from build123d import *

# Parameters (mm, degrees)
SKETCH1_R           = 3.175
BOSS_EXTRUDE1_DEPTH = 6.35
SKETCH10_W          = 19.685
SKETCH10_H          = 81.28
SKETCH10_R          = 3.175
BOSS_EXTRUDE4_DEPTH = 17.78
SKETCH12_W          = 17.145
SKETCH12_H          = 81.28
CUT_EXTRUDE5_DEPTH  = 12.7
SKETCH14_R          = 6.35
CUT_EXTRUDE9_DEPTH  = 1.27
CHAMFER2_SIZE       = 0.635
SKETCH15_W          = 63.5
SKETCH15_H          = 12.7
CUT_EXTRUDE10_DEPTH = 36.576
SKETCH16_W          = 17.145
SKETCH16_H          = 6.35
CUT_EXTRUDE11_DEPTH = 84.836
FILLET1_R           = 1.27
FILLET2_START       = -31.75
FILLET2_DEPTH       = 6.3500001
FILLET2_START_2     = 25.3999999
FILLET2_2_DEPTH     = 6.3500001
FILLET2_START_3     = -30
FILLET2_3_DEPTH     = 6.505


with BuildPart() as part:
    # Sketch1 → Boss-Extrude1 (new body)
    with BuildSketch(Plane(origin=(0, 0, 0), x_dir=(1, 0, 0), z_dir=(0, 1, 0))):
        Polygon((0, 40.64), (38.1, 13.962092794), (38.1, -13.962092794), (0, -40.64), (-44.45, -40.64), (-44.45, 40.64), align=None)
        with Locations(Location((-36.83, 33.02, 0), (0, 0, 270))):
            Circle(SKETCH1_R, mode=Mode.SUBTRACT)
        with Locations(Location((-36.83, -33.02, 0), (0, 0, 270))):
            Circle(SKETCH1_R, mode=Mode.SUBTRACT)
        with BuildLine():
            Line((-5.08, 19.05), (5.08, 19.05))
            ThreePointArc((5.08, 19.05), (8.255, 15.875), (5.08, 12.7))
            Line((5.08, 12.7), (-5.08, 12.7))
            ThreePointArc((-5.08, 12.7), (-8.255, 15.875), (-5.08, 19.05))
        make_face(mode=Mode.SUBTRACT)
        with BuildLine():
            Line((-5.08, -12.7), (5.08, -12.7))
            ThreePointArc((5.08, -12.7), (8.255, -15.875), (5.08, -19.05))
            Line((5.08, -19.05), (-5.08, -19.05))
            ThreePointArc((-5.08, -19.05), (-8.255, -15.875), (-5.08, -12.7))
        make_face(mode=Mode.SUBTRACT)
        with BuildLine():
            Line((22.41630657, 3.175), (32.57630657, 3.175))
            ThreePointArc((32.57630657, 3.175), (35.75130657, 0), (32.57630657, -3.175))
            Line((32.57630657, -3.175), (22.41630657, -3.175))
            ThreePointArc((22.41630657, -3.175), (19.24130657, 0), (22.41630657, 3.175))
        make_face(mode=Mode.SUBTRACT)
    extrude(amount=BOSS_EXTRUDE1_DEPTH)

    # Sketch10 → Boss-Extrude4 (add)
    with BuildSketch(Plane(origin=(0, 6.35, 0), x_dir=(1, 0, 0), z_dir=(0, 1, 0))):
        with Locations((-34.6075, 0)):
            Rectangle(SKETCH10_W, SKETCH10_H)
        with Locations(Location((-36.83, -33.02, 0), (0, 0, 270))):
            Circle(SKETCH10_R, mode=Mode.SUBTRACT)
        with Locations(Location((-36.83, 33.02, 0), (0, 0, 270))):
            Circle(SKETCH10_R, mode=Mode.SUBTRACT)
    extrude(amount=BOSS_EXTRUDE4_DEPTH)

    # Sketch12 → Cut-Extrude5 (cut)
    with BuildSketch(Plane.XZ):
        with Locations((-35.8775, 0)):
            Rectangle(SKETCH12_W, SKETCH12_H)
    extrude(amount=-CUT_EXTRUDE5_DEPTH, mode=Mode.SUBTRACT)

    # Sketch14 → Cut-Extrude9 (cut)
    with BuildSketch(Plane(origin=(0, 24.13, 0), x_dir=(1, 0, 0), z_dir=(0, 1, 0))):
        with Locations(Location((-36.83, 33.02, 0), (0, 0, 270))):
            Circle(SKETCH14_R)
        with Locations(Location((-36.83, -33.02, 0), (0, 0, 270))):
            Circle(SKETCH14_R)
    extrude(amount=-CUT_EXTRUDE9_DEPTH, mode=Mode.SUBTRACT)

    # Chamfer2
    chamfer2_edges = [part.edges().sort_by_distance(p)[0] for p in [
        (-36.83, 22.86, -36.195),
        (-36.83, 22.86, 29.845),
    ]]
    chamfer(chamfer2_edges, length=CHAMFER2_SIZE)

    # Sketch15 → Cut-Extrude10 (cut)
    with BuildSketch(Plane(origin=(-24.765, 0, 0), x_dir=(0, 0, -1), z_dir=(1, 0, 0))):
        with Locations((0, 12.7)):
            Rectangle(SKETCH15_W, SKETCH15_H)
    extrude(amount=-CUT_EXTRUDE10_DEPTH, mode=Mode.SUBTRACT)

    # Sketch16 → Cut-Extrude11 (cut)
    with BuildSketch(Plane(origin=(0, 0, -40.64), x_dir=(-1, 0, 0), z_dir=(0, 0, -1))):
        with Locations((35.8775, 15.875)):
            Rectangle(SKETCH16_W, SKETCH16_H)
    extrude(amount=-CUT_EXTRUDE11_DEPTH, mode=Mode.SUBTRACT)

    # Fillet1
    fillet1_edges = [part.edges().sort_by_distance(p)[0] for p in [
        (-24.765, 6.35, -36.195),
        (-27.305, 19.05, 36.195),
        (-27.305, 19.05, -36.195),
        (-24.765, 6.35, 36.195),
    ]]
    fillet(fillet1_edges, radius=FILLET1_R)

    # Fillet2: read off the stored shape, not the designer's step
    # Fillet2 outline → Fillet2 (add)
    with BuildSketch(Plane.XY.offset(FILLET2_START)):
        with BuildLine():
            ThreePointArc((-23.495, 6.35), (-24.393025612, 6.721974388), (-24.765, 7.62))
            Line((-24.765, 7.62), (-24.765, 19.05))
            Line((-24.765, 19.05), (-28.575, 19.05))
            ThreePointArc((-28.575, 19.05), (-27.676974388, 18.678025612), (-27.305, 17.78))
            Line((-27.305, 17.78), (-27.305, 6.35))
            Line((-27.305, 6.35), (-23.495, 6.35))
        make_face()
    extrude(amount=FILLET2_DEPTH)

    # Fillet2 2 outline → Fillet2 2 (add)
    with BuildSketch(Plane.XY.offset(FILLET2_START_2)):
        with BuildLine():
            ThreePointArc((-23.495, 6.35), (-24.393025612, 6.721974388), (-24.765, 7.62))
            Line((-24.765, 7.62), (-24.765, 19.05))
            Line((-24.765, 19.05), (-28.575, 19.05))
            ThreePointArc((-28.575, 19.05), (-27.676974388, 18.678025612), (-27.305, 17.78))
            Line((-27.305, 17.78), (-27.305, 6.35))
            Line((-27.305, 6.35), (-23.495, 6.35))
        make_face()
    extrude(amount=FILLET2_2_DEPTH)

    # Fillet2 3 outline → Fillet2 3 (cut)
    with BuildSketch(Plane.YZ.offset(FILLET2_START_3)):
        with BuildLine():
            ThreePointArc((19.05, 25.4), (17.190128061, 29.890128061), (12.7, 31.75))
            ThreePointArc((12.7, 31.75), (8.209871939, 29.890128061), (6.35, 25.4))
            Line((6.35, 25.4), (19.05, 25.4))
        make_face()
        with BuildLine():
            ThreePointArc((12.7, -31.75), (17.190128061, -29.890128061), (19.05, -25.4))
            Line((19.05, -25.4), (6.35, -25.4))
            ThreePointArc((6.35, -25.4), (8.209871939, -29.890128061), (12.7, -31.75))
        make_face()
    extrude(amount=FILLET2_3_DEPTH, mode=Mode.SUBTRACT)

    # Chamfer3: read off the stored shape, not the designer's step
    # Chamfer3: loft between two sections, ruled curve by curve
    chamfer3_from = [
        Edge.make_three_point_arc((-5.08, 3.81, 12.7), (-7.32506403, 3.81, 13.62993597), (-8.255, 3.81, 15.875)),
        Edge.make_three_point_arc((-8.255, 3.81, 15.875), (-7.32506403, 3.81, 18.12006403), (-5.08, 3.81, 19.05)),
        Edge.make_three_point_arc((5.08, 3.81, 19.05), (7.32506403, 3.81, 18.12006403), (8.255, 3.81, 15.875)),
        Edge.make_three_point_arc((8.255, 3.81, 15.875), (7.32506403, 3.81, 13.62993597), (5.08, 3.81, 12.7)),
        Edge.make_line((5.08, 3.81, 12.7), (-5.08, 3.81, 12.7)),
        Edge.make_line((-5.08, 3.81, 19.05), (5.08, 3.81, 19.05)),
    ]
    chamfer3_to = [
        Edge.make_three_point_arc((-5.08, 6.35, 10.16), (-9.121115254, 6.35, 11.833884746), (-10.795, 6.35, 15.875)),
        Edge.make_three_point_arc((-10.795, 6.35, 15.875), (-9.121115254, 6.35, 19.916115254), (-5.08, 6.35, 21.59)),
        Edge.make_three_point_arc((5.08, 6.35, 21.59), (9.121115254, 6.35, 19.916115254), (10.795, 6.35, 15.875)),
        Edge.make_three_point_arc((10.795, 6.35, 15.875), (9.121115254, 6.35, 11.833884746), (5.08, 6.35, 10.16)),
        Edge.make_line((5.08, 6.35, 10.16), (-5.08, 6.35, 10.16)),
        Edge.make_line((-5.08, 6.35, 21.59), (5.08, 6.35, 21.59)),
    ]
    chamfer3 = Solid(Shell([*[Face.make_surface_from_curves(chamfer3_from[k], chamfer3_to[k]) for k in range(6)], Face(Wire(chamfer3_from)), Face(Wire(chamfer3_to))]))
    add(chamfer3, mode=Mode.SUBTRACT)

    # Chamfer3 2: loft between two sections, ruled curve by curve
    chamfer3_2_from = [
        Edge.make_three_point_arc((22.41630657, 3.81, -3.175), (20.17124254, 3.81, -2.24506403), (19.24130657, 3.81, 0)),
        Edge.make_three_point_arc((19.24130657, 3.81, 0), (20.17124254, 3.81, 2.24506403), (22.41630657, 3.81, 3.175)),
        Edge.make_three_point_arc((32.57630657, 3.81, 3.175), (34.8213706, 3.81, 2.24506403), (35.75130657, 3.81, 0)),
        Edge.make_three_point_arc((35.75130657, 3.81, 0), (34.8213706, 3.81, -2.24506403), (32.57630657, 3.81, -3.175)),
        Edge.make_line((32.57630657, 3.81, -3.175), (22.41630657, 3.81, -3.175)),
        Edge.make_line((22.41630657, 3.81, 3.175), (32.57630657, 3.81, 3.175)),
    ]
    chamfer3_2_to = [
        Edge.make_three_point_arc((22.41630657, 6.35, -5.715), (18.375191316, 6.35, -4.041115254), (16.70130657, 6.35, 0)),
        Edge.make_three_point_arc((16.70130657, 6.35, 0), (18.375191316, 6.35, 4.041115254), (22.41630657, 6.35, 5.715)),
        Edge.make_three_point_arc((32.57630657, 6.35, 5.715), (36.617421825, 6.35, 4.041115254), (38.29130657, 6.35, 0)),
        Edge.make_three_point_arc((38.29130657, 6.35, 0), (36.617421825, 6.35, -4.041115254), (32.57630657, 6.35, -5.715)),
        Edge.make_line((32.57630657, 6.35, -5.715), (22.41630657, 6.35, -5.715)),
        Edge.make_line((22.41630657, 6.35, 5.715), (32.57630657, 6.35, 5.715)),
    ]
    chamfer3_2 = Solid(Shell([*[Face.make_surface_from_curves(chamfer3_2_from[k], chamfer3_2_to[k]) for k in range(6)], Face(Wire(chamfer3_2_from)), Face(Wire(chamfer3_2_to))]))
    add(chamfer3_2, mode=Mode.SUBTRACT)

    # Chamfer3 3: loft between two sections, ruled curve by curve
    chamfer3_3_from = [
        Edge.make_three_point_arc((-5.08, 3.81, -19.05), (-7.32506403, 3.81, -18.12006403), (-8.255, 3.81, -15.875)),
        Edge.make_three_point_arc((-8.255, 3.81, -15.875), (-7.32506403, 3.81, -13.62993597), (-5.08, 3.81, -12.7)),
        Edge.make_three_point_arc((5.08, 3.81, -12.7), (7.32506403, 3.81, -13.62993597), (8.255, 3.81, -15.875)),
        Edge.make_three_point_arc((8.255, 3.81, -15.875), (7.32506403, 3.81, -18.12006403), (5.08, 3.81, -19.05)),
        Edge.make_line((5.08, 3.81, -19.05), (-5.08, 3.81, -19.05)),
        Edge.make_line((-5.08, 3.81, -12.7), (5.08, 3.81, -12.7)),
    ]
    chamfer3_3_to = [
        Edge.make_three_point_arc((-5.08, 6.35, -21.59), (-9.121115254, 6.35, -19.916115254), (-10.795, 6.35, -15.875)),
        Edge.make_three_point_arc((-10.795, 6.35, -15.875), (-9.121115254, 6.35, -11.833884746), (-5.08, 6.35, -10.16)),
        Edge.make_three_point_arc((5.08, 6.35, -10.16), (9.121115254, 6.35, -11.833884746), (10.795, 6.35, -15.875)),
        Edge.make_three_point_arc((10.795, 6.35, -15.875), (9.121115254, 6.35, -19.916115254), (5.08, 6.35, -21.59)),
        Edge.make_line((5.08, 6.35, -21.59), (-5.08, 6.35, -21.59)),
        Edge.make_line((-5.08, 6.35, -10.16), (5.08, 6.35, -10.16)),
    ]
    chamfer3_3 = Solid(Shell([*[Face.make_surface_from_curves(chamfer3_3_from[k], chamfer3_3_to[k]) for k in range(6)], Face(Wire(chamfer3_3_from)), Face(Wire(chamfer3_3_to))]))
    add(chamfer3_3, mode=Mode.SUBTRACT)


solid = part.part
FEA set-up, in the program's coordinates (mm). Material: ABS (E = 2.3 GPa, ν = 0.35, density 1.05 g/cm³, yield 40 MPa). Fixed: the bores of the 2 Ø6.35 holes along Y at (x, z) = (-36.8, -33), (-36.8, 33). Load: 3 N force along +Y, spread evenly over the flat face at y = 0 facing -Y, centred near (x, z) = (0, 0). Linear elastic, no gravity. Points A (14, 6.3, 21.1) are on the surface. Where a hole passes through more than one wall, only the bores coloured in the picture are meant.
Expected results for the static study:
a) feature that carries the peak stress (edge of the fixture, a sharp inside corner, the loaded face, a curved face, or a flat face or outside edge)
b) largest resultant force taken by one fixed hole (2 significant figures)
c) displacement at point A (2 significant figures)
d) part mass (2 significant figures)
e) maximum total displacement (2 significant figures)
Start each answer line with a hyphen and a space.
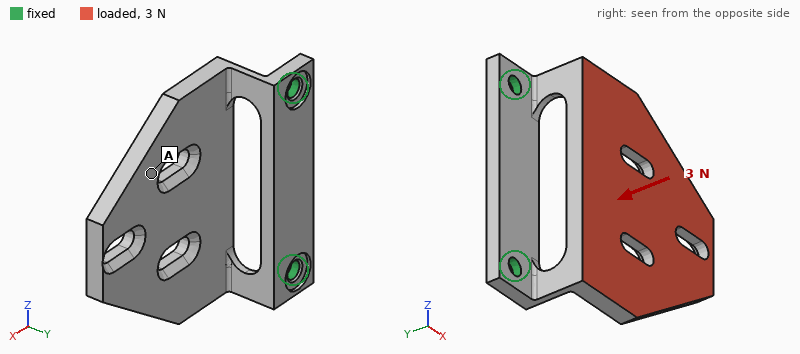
- a curved face
- 1.5 N
- 0.79 mm
- 35 g
- 1.3 mm
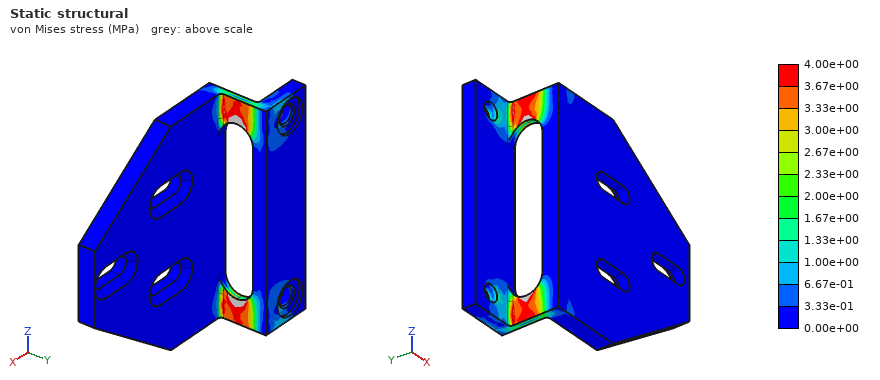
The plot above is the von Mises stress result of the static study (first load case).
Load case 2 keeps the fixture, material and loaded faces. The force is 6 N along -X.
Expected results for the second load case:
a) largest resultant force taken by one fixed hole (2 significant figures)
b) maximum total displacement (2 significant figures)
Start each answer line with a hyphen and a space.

- 3.0 N
- 1.2 mm
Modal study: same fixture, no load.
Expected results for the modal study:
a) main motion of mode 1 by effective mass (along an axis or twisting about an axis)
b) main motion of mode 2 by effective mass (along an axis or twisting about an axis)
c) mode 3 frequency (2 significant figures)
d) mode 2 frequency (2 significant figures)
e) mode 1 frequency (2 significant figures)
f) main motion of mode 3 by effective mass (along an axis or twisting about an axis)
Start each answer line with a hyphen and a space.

- along Y
- along Z
- 450 Hz
- 370 Hz
- 60 Hz
- along X
